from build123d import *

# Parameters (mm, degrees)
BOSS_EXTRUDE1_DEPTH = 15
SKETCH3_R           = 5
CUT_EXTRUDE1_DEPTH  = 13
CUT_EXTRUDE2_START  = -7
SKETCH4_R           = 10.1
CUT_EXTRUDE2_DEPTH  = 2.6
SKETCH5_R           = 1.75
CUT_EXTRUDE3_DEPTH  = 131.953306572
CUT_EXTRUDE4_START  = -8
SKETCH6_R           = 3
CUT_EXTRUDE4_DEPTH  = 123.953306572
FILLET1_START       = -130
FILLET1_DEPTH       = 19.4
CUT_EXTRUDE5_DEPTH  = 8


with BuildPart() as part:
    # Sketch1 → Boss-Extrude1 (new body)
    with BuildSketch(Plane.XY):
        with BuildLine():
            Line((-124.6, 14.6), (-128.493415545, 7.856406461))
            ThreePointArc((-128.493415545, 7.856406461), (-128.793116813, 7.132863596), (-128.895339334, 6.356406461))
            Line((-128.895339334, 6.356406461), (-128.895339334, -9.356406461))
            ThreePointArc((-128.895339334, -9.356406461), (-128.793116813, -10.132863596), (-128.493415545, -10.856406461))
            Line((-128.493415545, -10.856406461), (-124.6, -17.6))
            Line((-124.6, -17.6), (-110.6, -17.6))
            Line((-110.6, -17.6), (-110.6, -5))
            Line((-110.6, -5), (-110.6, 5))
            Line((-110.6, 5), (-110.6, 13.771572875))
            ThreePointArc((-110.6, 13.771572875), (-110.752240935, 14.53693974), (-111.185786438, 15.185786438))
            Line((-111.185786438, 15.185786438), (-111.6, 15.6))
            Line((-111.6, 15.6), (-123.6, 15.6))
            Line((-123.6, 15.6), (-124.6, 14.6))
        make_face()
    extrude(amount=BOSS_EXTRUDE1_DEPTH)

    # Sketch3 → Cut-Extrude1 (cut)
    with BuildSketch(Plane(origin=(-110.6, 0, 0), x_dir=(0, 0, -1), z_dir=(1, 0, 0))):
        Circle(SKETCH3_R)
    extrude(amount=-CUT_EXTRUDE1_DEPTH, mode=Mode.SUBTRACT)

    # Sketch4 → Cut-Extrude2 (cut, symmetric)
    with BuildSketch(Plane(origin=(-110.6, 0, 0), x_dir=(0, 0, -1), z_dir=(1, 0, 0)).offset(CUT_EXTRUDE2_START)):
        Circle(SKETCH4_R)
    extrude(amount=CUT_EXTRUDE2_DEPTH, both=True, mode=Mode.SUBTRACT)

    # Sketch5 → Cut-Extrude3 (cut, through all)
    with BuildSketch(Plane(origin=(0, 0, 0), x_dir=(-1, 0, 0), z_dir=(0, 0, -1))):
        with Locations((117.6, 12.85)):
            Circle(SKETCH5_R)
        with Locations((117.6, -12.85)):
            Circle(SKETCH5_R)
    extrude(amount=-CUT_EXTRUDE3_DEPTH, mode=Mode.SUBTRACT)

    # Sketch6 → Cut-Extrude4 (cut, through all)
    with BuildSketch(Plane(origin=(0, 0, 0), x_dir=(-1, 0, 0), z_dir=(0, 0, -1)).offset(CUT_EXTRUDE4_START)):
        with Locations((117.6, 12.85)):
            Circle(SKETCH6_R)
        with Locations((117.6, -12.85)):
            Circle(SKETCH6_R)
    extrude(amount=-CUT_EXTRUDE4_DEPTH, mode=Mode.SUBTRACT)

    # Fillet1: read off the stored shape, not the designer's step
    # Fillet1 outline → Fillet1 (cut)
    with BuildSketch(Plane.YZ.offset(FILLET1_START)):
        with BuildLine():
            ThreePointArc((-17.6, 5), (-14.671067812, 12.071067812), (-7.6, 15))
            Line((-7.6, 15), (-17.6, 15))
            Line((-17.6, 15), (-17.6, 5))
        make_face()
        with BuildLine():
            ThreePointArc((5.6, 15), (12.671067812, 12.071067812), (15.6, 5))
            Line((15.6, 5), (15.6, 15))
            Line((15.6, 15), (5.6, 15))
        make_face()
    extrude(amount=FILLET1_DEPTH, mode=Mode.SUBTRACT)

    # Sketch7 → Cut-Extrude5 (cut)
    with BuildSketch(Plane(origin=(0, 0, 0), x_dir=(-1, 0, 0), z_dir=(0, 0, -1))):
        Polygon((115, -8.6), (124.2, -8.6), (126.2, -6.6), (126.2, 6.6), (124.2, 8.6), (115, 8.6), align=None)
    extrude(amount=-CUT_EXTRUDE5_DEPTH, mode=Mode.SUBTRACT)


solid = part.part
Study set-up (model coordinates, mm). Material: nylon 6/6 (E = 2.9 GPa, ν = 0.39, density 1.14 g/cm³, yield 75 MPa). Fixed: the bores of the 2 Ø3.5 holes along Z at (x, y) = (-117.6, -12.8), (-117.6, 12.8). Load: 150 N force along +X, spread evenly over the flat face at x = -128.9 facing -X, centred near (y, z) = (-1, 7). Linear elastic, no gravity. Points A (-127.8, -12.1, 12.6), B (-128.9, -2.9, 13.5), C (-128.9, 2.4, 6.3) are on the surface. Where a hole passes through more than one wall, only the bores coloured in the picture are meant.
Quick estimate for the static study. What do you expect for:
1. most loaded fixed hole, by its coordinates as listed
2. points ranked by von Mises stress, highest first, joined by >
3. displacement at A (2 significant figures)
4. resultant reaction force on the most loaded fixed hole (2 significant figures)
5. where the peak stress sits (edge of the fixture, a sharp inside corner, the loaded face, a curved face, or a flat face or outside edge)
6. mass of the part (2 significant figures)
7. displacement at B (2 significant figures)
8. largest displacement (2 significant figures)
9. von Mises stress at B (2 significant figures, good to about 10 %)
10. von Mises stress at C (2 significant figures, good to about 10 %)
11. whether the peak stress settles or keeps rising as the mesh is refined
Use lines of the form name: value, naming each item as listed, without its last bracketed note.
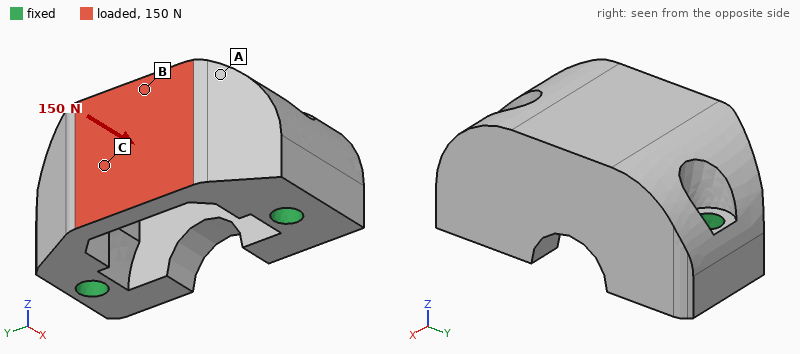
most loaded fixed hole, by its coordinates as listed: (-117.6, -12.8)
points ranked by von Mises stress, highest first, joined by >: C > B > A
displacement at A: 9.1 µm
resultant reaction force on the most loaded fixed hole: 88 N
where the peak stress sits: edge of the fixture
mass of the part: 6.5 g
displacement at B: 14 µm
largest displacement: 38 µm
von Mises stress at B: 1.1 MPa
von Mises stress at C: 2.8 MPa
whether the peak stress settles or keeps rising as the mesh is refined: keeps rising
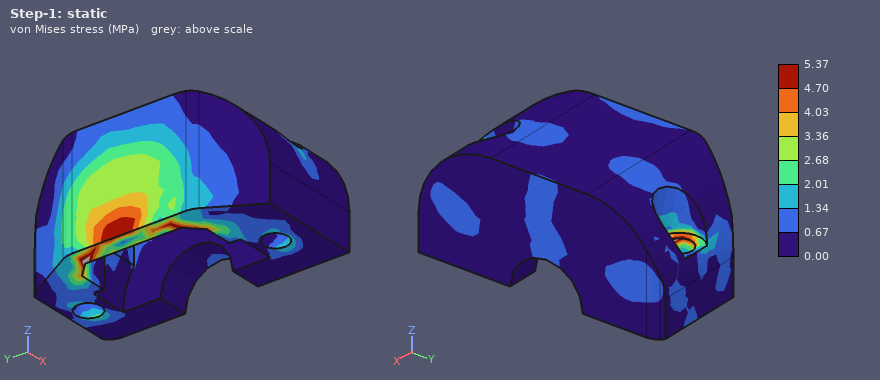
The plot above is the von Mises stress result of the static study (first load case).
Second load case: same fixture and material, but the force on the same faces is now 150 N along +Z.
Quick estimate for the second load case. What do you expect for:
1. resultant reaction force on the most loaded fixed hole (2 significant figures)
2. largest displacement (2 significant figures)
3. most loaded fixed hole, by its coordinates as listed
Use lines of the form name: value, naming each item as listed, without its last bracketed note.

resultant reaction force on the most loaded fixed hole: 94 N
largest displacement: 60 µm
most loaded fixed hole, by its coordinates as listed: (-117.6, -12.8)
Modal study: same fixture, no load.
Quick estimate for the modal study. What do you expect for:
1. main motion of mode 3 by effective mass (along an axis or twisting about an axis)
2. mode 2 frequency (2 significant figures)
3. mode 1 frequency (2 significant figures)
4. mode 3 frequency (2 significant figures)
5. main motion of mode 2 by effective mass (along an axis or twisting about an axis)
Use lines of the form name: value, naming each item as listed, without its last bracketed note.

main motion of mode 3 by effective mass: along Z
mode 2 frequency: 10 kHz
mode 1 frequency: 6500 Hz
mode 3 frequency: 11 kHz
main motion of mode 2 by effective mass: along Y
